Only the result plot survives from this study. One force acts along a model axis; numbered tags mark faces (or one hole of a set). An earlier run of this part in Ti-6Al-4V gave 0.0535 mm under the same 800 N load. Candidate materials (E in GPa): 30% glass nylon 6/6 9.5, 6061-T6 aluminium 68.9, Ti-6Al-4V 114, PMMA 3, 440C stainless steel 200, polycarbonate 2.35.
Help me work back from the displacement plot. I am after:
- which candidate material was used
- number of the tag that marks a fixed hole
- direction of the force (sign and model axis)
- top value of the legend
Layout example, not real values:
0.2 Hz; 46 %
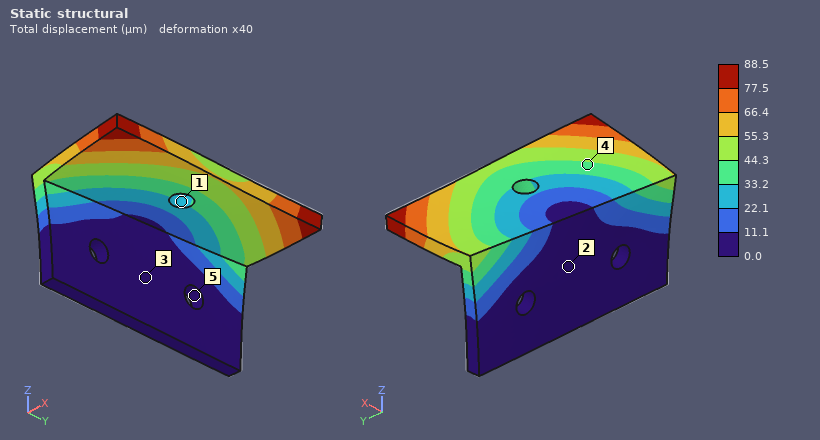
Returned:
6061-T6 aluminium; 5; -Y; 88.5 µm
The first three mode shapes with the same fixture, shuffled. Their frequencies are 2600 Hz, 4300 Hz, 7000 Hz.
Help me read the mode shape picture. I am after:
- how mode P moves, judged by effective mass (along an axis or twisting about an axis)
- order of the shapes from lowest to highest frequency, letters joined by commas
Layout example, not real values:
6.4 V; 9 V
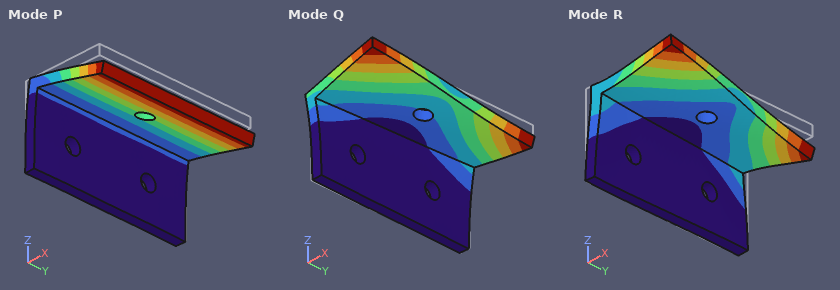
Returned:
along Z; P, Q, R
